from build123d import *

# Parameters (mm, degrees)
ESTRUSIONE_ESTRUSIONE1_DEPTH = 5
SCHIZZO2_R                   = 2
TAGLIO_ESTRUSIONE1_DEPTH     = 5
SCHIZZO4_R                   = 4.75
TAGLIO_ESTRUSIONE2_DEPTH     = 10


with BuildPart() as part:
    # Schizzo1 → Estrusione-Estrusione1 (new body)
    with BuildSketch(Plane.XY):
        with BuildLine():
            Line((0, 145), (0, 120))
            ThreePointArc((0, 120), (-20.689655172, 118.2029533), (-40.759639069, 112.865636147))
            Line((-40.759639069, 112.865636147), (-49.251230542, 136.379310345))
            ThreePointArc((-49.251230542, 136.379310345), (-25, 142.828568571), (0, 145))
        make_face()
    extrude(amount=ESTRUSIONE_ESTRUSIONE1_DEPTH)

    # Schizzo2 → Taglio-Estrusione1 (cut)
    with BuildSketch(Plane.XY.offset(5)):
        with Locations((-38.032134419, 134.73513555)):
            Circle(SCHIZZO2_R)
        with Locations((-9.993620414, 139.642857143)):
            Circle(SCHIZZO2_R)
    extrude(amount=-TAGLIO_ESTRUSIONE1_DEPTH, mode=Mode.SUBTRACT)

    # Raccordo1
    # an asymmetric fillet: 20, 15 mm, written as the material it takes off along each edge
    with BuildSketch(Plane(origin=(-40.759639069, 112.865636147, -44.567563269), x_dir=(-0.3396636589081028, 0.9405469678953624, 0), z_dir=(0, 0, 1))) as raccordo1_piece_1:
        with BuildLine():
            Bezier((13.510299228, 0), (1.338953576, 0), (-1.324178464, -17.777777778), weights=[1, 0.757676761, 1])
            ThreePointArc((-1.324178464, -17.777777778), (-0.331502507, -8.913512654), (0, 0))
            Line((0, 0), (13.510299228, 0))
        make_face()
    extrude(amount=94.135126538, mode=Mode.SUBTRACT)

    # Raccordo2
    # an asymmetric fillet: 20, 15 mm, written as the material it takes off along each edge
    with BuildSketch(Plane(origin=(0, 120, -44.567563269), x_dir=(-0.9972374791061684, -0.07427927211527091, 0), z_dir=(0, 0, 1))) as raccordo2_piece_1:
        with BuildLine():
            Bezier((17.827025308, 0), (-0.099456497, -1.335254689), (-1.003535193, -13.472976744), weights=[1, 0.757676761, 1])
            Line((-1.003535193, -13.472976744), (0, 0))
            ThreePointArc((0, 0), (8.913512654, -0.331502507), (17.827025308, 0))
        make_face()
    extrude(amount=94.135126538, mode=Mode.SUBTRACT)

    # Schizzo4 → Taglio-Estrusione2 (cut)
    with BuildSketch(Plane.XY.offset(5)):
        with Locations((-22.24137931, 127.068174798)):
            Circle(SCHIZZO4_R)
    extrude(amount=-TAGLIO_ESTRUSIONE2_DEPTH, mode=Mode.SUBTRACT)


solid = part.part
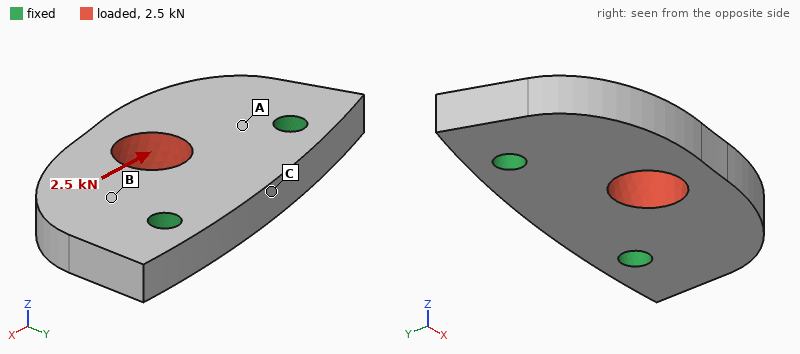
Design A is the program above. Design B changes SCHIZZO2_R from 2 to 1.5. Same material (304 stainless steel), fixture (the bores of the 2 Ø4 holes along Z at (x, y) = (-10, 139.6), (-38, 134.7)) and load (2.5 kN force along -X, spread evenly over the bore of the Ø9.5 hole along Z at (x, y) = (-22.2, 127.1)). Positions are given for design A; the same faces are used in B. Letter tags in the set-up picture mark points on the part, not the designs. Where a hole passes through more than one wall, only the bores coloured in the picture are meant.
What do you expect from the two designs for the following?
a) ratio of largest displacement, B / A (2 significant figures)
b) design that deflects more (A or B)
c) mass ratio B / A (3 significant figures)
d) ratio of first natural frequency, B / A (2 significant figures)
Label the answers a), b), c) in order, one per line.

a) 1.1
b) B
c) 1.01
d) 0.92
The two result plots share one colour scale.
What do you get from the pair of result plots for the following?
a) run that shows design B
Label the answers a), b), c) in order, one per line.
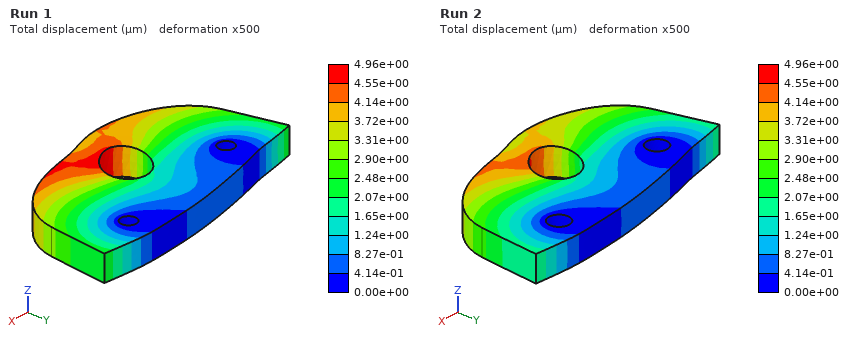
a) Run 1
